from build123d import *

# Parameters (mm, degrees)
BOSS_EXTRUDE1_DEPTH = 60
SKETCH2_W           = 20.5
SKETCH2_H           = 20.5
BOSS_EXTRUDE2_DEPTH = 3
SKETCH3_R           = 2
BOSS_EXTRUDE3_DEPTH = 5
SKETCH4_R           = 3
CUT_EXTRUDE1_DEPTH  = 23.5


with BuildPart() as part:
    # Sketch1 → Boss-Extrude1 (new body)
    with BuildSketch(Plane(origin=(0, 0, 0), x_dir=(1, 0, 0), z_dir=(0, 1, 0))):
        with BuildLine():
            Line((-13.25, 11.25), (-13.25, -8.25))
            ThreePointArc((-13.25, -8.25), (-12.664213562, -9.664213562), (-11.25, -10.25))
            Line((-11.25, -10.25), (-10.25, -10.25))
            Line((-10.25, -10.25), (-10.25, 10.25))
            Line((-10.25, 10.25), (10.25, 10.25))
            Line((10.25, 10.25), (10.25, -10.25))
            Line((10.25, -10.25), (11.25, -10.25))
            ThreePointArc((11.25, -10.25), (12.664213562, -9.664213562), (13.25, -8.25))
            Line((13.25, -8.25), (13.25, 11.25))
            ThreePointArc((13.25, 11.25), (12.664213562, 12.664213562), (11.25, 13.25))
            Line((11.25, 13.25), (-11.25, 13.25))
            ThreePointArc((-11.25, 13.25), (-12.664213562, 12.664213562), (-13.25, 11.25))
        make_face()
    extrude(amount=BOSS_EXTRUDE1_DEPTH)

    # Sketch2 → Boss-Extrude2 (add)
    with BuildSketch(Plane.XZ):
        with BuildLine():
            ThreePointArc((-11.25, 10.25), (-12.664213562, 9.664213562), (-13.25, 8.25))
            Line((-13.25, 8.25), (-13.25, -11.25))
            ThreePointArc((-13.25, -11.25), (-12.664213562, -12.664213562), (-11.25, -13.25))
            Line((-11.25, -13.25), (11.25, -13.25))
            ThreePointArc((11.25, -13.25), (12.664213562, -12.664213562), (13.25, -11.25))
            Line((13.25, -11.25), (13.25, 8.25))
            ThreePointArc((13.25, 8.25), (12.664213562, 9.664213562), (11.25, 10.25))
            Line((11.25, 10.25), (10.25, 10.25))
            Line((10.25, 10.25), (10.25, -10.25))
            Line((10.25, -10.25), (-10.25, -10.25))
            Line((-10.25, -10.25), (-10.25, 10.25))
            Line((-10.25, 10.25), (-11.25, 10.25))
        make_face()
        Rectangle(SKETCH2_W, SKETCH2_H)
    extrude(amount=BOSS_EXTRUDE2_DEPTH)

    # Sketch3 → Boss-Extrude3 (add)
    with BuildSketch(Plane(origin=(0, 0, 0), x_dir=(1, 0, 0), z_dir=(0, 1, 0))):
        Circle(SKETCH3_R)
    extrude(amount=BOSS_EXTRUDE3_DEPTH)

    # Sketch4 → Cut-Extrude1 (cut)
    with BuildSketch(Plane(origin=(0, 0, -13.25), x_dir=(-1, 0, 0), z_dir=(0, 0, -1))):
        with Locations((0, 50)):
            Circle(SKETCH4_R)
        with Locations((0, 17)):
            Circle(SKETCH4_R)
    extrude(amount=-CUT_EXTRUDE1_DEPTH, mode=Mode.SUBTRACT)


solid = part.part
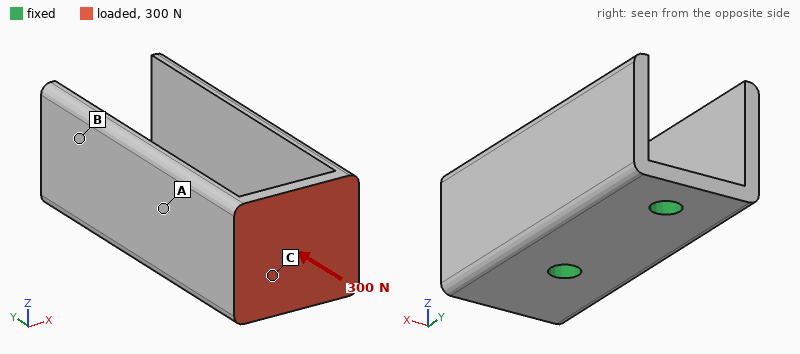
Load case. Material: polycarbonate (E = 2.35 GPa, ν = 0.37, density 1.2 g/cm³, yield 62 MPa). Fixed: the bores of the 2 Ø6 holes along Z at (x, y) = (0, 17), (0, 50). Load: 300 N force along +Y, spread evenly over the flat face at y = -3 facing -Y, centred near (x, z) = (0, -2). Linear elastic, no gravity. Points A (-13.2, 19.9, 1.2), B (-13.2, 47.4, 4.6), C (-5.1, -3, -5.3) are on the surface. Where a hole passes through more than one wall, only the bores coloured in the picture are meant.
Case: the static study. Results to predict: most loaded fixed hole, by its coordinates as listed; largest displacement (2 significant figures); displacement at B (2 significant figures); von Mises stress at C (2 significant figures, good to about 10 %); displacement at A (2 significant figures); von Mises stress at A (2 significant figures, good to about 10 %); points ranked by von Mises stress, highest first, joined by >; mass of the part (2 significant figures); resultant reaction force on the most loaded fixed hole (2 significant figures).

(0, 17)
0.36 mm
0.19 mm
4.7 MPa
0.094 mm
2.3 MPa
C > A > B
16 g
200 N
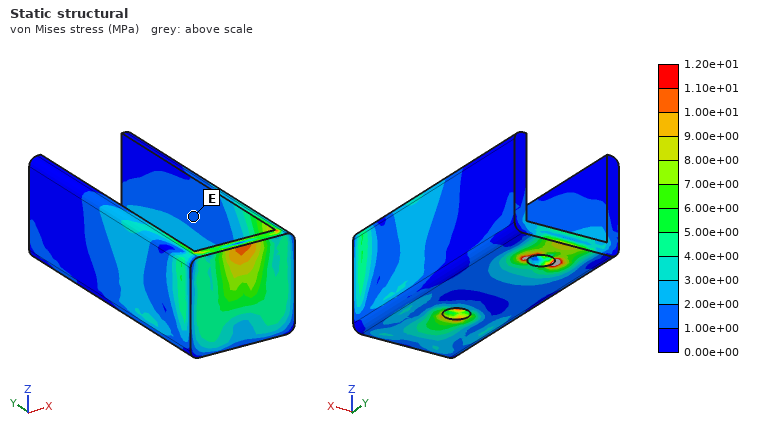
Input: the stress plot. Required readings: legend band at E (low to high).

1.00e+00 to 2.00e+00 MPa
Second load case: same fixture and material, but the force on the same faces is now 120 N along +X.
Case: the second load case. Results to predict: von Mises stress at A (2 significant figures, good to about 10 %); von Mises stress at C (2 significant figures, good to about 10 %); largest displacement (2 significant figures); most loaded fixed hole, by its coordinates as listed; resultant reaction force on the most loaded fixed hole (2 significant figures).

2.3 MPa
2.1 MPa
0.74 mm
(0, 17)
170 N
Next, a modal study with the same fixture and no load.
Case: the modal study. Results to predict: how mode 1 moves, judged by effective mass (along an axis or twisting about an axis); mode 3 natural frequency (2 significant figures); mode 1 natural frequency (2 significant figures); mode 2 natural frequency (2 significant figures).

along X
1200 Hz
790 Hz
1000 Hz
